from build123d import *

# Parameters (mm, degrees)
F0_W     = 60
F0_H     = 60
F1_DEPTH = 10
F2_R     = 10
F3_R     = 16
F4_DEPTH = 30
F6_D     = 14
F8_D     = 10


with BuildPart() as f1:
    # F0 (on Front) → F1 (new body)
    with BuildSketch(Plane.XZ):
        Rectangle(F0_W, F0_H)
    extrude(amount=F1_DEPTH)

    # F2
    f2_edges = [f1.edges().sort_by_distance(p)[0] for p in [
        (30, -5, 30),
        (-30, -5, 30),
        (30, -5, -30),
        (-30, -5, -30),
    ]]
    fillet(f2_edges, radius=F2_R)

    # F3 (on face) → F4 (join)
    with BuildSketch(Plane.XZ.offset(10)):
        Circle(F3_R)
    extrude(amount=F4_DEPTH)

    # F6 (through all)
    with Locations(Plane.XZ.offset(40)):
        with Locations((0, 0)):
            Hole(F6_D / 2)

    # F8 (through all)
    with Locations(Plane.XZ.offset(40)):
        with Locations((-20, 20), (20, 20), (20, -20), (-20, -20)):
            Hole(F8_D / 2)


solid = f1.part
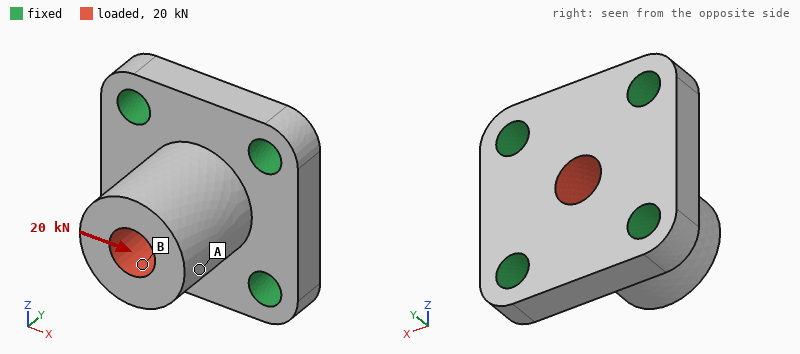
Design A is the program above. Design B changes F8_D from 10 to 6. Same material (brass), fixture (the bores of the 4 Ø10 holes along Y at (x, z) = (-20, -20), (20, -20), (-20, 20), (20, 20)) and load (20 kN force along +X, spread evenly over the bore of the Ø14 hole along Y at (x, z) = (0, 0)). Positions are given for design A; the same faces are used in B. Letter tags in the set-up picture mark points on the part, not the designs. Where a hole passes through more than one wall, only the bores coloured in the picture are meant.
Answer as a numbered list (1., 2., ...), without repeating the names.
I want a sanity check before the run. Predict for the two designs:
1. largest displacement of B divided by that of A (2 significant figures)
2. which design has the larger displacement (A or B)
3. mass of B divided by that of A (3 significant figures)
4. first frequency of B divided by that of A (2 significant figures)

1. 1.2
2. B
3. 1.04
4. 0.92
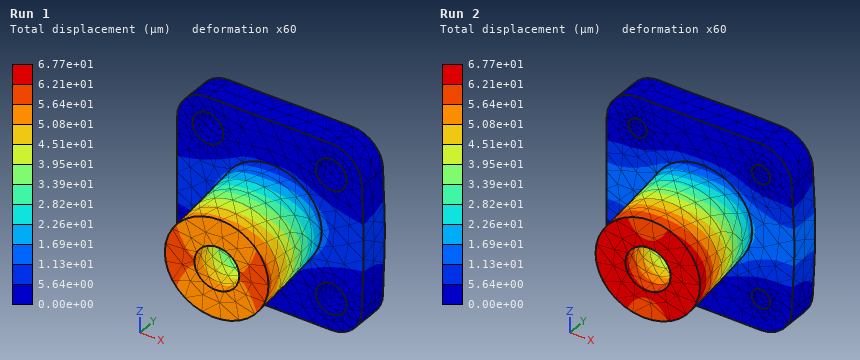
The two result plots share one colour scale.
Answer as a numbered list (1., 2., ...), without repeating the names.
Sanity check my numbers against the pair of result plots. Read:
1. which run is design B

1. Run 2
